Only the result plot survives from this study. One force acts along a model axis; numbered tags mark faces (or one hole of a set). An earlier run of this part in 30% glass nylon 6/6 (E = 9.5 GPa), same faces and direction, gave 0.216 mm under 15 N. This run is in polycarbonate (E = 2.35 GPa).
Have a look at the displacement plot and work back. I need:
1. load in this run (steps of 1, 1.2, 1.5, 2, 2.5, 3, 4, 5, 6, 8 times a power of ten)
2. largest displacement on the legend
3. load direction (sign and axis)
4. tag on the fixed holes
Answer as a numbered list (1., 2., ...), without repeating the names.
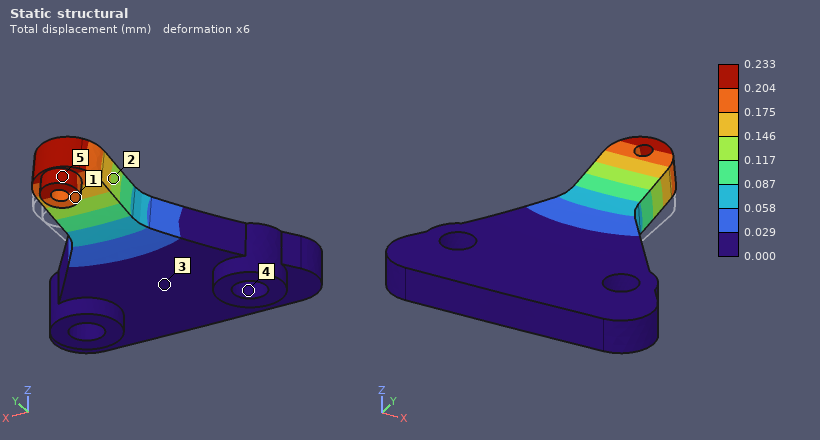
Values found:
1. 4 N
2. 0.233 mm
3. +Z
4. 4
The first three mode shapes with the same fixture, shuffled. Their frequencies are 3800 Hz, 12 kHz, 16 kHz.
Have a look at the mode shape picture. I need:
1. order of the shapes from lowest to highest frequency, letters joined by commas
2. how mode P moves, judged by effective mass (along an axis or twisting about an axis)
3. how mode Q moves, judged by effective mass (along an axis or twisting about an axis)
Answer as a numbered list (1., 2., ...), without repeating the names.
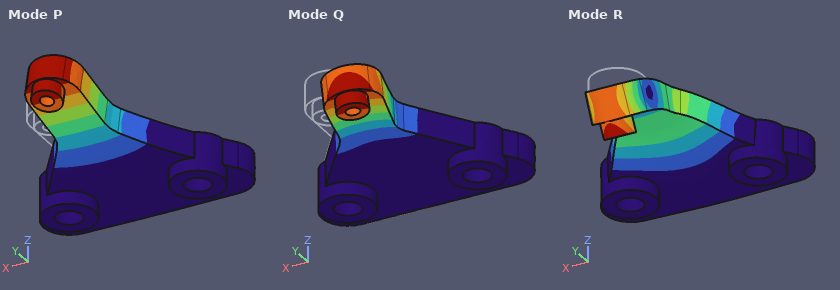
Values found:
1. P, Q, R
2. along Z
3. along X
